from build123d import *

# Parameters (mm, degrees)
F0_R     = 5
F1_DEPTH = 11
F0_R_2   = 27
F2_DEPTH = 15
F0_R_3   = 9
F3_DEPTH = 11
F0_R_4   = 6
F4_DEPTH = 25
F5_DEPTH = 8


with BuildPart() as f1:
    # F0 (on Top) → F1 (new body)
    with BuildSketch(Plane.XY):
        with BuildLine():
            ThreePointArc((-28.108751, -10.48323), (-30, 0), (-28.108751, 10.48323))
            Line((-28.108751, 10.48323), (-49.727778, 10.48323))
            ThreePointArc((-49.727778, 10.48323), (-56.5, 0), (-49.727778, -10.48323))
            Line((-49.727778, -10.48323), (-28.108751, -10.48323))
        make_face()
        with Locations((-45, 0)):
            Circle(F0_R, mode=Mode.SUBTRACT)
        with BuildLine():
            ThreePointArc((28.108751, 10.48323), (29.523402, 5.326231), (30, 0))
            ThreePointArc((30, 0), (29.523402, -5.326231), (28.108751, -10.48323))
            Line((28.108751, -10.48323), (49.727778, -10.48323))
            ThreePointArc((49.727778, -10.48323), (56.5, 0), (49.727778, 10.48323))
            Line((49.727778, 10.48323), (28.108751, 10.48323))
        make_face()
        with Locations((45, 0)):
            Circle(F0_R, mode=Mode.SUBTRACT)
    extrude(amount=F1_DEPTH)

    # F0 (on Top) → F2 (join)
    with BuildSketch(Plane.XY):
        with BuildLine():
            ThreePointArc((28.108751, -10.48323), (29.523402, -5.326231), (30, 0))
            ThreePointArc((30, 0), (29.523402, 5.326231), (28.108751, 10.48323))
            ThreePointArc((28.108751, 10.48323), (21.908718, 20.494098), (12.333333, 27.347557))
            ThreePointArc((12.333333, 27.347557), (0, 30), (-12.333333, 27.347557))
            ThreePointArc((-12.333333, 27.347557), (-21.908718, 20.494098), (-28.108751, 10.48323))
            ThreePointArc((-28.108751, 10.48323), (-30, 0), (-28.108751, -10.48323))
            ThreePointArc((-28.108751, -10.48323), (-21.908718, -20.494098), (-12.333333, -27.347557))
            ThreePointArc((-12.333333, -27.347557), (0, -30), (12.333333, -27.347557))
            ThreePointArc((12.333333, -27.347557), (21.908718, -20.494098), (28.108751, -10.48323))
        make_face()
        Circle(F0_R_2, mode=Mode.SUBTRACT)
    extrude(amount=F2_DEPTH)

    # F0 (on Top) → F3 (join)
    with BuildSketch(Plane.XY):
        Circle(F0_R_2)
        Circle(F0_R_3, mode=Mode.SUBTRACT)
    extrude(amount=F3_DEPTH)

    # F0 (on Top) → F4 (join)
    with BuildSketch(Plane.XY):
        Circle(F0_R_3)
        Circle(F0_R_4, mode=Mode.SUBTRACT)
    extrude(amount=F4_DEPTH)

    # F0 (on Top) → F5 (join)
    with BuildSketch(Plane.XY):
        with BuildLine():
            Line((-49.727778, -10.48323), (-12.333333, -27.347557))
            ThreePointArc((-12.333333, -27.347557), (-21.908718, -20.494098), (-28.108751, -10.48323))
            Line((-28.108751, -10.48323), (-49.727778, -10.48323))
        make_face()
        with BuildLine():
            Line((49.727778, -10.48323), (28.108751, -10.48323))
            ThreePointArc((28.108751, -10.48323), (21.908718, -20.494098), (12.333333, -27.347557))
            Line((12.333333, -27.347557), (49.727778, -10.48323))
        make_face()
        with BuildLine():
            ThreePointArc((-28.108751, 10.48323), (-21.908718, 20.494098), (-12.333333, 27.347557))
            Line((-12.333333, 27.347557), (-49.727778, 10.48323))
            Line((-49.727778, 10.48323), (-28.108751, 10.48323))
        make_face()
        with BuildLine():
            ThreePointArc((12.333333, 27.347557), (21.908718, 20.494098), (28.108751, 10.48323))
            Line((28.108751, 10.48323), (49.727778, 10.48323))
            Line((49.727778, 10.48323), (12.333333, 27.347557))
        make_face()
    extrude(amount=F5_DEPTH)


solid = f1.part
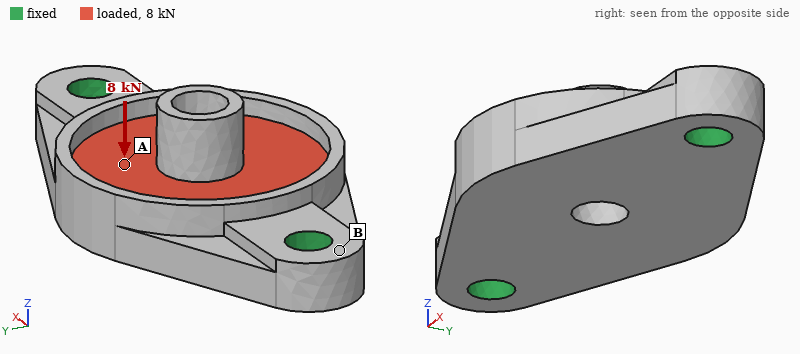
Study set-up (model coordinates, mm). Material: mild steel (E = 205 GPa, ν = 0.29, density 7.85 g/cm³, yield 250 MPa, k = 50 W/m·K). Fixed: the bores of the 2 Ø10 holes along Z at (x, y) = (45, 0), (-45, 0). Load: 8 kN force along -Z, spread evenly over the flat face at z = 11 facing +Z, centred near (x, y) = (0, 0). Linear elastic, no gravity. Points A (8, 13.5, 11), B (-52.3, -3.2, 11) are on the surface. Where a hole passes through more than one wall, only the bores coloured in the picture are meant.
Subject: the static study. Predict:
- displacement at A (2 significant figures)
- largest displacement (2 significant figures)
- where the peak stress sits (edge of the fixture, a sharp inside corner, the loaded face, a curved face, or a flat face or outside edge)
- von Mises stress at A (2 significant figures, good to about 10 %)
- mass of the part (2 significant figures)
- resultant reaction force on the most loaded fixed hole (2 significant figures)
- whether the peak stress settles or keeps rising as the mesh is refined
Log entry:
27 µm
33 µm
edge of the fixture
46 MPa
380 g
4.0 kN
keeps rising
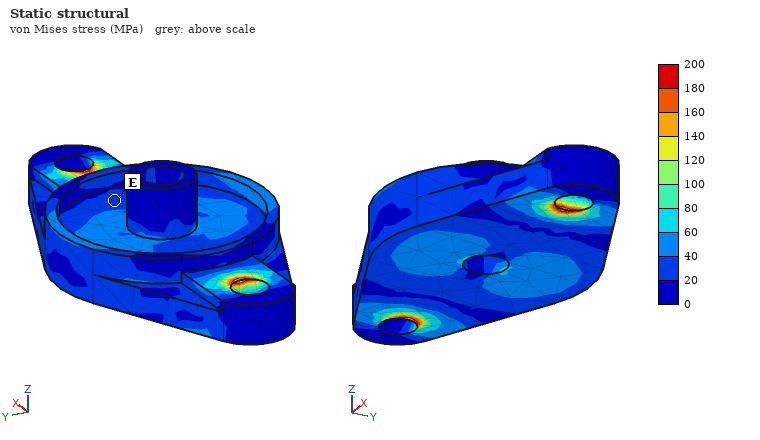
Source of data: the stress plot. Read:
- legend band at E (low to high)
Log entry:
20 to 40 MPa
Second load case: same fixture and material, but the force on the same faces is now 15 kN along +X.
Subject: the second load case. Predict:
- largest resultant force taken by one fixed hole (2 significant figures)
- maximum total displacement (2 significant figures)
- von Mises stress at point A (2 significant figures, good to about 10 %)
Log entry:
7.6 kN
5.5 µm
17 MPa
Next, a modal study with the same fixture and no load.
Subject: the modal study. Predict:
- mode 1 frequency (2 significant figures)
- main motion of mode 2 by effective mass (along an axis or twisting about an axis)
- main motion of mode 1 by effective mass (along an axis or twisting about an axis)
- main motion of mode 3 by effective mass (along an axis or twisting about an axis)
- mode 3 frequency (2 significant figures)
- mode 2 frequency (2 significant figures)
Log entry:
5200 Hz
along Z
twisting about X
along Y
11 kHz
5400 Hz
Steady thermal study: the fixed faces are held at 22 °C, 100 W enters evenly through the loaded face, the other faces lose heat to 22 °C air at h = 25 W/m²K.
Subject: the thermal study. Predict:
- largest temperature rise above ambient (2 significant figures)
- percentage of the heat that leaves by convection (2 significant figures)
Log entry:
74 K
14 %
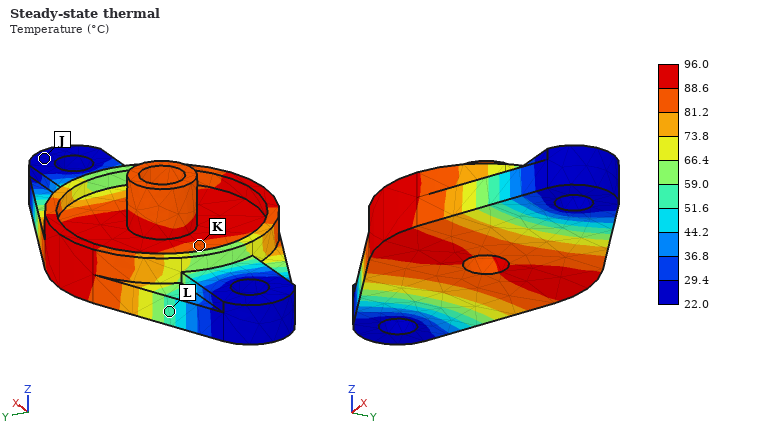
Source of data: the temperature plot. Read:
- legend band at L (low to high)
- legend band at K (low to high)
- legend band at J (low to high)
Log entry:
51.6 to 59.0 °C
81.2 to 88.6 °C
22.0 to 29.4 °C
